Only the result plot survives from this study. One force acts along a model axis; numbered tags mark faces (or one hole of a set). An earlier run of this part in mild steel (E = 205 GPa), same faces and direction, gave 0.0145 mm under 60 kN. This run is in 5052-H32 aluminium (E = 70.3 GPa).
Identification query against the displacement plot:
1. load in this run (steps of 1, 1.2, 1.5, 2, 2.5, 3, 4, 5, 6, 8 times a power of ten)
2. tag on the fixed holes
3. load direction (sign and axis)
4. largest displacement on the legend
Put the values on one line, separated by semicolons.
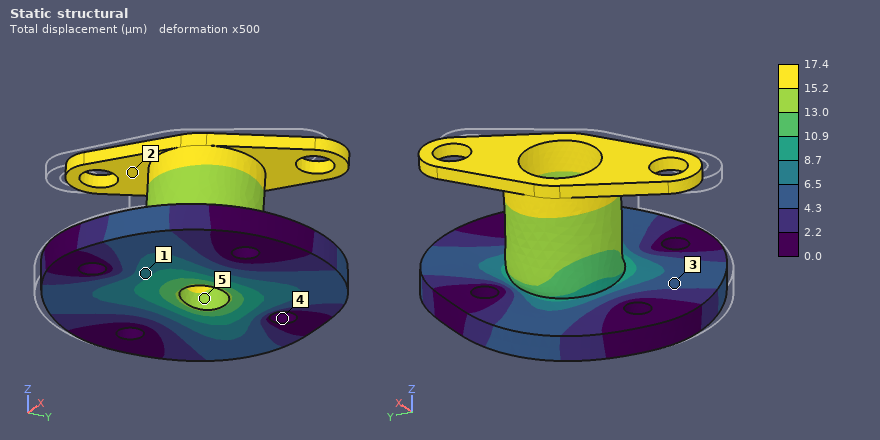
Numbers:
25 kN; 4; +Y; 17.4 µm
